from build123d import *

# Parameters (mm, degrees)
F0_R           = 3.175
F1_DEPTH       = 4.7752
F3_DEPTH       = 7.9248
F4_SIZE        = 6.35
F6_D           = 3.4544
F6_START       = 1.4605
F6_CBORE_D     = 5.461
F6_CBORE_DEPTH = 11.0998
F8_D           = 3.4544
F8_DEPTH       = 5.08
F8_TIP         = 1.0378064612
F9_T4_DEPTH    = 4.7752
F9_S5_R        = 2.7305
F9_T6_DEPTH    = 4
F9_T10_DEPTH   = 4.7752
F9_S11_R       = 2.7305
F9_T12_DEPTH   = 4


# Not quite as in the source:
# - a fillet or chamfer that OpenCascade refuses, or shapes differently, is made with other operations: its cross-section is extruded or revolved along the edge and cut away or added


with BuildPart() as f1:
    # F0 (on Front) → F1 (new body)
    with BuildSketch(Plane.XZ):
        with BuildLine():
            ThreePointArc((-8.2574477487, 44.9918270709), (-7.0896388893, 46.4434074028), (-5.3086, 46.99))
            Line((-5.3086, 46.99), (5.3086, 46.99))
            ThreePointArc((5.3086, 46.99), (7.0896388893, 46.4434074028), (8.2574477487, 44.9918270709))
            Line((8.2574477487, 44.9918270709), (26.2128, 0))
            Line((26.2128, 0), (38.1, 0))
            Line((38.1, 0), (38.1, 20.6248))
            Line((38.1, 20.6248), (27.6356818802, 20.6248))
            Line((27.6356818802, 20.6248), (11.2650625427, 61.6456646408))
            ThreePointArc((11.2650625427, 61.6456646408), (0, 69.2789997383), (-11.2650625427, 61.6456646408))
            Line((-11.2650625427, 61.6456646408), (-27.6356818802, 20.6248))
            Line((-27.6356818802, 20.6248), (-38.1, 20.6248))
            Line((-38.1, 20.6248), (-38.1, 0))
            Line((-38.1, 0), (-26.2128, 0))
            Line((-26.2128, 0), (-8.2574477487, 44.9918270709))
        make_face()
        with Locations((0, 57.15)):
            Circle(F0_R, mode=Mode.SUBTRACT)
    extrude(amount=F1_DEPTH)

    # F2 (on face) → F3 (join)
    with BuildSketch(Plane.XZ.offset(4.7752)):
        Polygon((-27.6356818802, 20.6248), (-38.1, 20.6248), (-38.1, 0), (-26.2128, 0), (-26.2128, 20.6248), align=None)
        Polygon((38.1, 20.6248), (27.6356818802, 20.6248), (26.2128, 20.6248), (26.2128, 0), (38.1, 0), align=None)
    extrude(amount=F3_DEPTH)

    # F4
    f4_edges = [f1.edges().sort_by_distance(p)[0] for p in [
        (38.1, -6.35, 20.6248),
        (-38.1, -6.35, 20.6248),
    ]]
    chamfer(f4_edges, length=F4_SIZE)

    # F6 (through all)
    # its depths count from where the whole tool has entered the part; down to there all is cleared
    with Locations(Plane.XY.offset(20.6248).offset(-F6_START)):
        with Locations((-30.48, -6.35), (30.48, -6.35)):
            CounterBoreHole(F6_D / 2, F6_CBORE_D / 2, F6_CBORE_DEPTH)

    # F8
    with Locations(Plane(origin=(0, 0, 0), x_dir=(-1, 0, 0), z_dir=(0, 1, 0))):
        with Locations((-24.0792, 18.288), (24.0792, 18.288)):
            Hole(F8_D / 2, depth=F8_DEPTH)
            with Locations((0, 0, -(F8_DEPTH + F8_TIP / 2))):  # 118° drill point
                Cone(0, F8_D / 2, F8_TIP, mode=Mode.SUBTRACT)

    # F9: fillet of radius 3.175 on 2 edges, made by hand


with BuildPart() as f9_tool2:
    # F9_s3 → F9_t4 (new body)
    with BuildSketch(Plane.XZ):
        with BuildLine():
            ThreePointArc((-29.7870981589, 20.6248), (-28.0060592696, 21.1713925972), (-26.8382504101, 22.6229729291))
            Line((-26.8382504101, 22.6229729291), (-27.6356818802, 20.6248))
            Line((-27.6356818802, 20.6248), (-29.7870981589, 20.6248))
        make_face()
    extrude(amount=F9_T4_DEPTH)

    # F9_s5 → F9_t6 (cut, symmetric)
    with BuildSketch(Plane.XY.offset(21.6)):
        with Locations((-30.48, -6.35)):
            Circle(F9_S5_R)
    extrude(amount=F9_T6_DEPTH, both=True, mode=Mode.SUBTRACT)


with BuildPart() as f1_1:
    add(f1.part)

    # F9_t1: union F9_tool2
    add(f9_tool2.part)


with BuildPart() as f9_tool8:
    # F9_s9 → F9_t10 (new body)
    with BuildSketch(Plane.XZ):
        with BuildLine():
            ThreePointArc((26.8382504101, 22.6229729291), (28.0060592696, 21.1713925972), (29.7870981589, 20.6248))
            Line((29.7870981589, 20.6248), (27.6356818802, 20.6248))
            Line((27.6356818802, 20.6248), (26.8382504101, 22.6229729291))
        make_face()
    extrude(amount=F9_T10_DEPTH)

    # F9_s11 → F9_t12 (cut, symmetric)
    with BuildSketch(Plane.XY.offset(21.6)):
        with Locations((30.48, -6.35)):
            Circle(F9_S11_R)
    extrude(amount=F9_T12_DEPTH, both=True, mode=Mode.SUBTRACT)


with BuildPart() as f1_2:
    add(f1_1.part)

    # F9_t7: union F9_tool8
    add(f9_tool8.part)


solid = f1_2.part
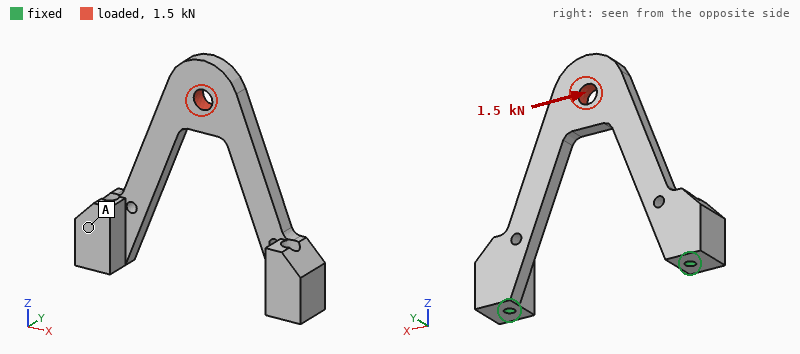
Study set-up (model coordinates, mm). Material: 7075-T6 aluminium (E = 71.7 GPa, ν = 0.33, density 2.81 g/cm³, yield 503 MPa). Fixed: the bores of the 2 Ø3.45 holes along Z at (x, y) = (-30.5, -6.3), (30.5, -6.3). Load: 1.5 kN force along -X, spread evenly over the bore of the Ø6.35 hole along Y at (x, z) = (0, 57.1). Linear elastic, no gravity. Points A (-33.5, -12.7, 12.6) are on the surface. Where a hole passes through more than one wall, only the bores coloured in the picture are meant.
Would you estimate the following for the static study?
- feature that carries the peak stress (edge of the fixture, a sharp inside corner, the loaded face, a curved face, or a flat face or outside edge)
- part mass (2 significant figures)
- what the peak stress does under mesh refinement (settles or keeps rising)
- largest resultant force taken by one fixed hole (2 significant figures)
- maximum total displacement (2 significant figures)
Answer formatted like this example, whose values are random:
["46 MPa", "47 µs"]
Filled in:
["edge of the fixture", "30 g", "keeps rising", "1.3 kN", "97 µm"]
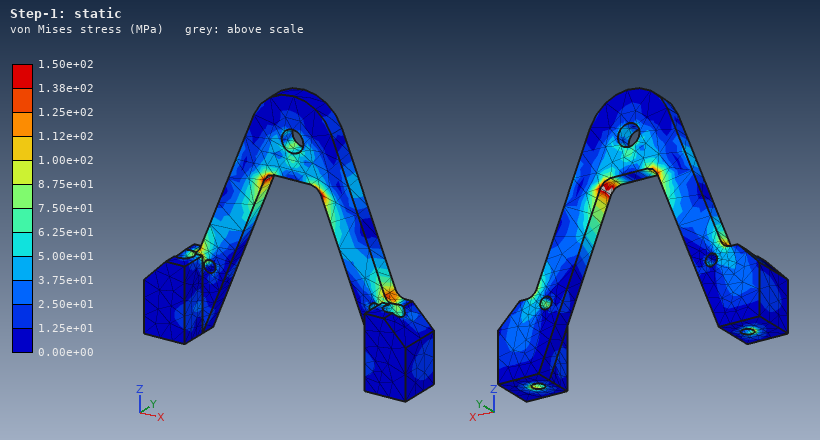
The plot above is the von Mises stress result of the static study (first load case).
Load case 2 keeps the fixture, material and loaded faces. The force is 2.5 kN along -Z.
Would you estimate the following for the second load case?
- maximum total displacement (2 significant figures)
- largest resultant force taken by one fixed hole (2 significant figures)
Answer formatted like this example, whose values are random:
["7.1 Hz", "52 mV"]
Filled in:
["57 µm", "1.4 kN"]
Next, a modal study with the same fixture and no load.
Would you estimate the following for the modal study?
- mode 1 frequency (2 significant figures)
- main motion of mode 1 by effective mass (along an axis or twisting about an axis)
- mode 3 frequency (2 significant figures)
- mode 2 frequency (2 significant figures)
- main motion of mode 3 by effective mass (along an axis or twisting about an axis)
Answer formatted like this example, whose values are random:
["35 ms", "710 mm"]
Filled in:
["1100 Hz", "along Y", "6000 Hz", "4700 Hz", "along X"]
